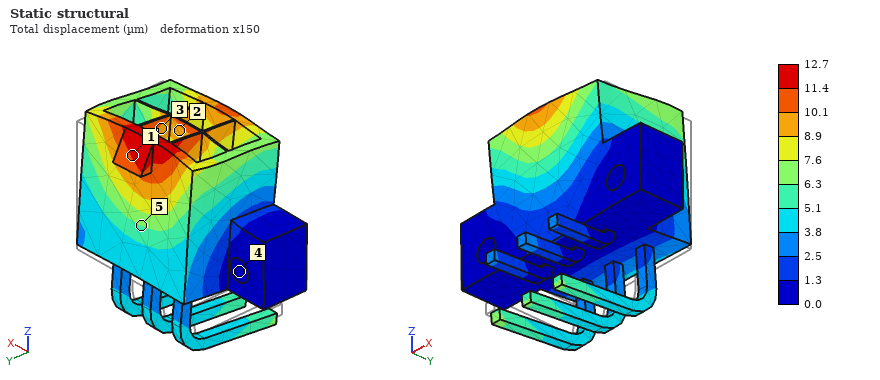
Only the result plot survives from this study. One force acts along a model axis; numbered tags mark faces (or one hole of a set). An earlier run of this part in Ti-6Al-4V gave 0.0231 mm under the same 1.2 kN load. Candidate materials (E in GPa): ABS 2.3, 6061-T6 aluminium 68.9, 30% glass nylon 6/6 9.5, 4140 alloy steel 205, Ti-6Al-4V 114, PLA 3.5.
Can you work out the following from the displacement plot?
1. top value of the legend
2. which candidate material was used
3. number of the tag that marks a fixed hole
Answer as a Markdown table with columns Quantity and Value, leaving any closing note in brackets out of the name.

| Quantity | Value |
|---|---|
| top value of the legend | 12.7 µm |
| which candidate material was used | 4140 alloy steel |
| number of the tag that marks a fixed hole | 4 |
